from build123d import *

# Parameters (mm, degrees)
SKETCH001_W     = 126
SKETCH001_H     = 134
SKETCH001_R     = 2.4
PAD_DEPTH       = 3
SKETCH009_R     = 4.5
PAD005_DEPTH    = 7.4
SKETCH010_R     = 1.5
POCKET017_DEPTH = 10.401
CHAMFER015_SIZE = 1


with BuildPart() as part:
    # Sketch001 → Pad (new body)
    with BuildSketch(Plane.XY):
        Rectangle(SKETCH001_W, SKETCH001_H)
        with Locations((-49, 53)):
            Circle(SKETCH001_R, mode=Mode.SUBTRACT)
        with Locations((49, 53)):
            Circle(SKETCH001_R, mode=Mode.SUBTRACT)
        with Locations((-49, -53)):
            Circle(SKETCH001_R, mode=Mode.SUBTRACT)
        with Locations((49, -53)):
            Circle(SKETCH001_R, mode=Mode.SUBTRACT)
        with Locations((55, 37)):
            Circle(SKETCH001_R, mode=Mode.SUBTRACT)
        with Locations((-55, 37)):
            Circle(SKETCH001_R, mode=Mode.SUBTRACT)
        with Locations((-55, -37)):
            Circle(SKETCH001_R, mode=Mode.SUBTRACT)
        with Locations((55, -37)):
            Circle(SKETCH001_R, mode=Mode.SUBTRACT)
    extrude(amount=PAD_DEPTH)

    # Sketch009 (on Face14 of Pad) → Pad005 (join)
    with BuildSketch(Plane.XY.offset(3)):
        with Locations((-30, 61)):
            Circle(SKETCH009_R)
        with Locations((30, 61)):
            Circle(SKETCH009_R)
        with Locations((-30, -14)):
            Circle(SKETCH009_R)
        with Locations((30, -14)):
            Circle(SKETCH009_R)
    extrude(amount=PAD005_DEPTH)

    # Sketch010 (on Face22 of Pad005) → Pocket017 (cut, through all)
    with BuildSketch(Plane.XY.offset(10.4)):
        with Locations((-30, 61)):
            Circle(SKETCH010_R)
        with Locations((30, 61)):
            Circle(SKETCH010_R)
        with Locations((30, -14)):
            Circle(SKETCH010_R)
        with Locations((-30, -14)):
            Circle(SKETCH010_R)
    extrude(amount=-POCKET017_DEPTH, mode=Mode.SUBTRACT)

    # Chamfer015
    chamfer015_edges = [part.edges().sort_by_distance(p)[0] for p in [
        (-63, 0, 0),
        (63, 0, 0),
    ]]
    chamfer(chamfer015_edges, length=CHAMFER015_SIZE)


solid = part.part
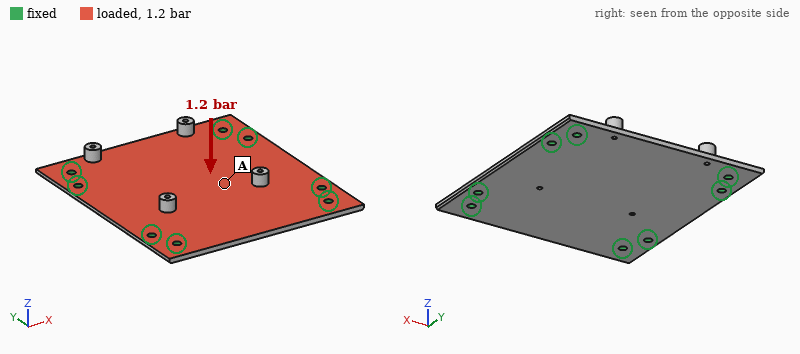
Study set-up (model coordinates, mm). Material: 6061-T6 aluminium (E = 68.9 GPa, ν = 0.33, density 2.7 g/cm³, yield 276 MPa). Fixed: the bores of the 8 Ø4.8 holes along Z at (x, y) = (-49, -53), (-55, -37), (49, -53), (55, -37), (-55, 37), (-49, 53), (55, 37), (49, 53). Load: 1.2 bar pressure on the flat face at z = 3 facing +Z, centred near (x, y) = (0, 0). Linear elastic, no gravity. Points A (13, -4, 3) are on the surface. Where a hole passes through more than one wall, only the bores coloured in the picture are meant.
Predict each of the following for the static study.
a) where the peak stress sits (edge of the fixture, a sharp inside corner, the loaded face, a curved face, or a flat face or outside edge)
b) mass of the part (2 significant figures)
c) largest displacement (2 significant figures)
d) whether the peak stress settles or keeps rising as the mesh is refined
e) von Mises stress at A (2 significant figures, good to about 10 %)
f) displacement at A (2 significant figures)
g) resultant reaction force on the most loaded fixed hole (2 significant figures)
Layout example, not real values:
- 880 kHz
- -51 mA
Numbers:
- edge of the fixture
- 140 g
- 0.36 mm
- keeps rising
- 33 MPa
- 0.33 mm
- 280 N
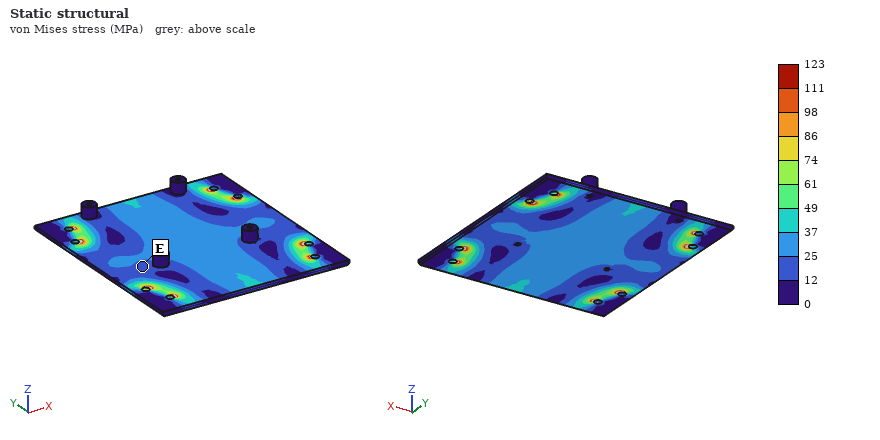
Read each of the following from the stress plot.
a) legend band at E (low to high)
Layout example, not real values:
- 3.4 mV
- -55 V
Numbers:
- 12 to 25 MPa
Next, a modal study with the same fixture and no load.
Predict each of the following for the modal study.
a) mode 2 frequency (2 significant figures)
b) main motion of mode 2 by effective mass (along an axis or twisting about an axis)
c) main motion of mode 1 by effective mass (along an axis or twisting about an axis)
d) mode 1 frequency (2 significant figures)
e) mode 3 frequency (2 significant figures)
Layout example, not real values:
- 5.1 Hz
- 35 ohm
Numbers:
- 1700 Hz
- twisting about X
- along Z
- 1200 Hz
- 2100 Hz
